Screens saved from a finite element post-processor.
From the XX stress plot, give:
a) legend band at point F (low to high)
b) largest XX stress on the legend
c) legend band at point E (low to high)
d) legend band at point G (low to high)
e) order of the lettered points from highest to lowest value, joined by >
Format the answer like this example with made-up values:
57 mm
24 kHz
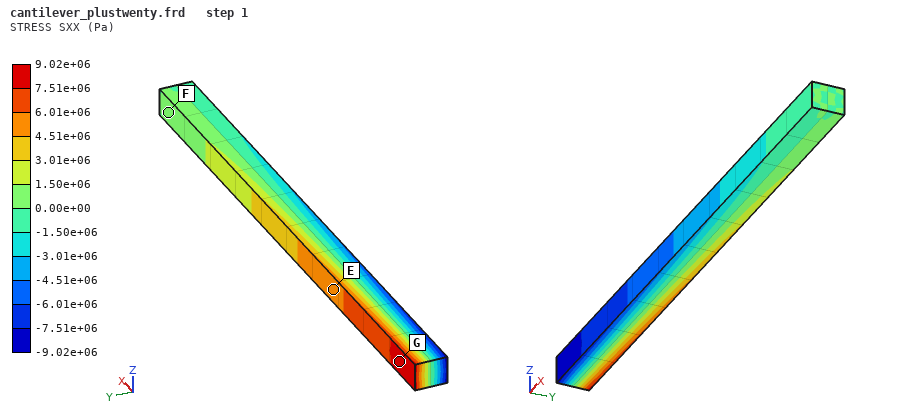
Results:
0.00e+00 to 1.50e+06 Pa
9.02e+06 Pa
4.51e+06 to 6.01e+06 Pa
7.51e+06 to 9.02e+06 Pa
G > E > F
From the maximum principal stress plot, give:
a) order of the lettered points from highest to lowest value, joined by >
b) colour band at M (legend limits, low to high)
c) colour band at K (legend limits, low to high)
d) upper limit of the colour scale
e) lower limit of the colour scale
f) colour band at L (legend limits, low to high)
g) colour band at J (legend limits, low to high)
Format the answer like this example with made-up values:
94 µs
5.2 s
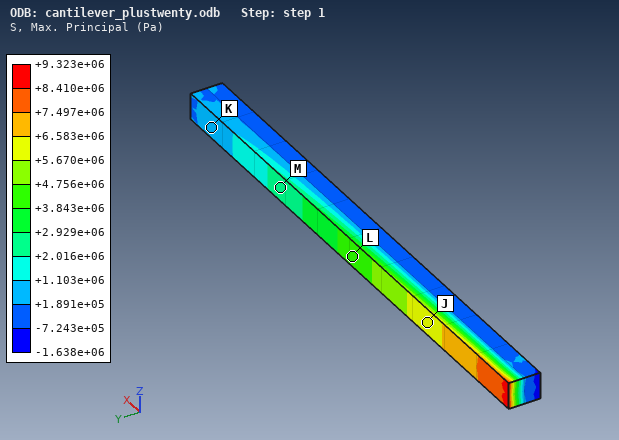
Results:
J > L > M > K
+2.016e+06 to +2.929e+06 Pa
+1.891e+05 to +1.103e+06 Pa
+9.323e+06 Pa
-1.638e+06 Pa
+3.843e+06 to +4.756e+06 Pa
+5.670e+06 to +6.583e+06 Pa
